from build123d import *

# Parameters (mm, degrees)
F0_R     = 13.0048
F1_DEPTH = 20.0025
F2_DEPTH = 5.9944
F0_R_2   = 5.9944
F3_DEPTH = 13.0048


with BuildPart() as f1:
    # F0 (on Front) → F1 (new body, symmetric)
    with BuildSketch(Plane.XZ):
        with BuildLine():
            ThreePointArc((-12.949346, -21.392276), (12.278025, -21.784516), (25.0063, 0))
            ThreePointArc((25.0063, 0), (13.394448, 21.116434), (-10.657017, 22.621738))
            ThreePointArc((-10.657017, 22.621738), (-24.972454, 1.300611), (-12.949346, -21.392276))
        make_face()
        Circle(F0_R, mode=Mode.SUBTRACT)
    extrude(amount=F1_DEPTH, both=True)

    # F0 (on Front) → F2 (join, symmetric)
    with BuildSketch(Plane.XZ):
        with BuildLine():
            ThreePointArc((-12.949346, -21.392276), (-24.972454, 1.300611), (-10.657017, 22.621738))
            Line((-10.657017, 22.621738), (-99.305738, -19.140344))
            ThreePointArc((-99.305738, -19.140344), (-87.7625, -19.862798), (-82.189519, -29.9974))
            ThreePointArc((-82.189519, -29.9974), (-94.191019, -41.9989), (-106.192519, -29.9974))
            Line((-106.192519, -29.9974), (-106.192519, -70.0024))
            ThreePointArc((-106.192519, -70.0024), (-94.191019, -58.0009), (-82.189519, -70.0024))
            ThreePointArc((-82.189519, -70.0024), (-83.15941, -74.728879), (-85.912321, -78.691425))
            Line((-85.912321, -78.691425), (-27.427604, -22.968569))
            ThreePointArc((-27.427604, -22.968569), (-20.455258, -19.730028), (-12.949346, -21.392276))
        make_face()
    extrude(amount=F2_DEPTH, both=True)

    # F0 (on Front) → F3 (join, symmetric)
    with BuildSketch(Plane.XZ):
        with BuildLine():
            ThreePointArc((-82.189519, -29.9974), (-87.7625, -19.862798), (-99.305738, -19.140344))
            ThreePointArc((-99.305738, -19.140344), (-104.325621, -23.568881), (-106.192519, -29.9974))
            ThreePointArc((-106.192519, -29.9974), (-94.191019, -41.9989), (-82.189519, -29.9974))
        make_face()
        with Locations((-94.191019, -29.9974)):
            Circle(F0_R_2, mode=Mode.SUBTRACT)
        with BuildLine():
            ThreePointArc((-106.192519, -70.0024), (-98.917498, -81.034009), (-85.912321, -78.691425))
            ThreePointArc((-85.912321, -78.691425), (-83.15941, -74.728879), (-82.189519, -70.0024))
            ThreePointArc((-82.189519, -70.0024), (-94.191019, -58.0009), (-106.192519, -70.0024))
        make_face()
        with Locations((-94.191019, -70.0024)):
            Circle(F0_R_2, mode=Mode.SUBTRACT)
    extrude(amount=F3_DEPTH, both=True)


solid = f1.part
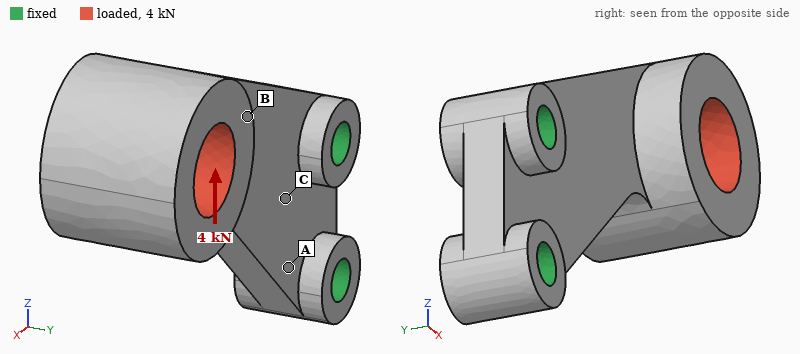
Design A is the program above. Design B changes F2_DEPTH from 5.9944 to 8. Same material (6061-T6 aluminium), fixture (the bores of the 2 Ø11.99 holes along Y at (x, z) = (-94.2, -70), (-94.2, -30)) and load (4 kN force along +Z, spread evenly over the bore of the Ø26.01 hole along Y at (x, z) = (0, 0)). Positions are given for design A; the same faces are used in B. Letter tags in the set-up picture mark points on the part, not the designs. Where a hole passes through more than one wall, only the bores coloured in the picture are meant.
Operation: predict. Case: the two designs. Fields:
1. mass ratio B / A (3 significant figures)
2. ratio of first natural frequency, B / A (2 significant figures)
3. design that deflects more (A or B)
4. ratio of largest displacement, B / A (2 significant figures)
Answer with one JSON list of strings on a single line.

["1.12", "1.5", "A", "0.77"]
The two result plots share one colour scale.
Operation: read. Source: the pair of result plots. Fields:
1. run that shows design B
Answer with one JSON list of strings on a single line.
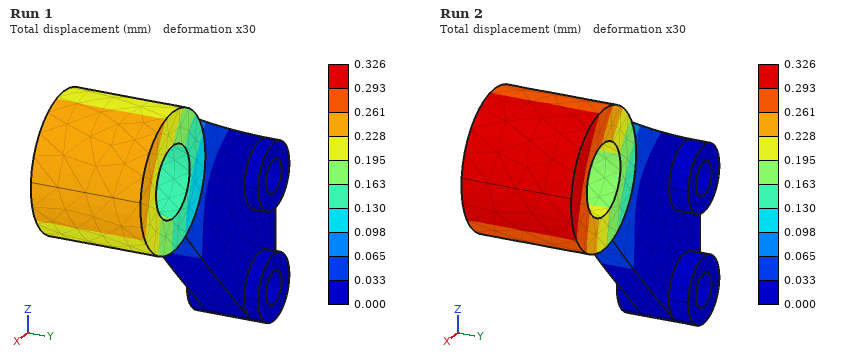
["Run 1"]
